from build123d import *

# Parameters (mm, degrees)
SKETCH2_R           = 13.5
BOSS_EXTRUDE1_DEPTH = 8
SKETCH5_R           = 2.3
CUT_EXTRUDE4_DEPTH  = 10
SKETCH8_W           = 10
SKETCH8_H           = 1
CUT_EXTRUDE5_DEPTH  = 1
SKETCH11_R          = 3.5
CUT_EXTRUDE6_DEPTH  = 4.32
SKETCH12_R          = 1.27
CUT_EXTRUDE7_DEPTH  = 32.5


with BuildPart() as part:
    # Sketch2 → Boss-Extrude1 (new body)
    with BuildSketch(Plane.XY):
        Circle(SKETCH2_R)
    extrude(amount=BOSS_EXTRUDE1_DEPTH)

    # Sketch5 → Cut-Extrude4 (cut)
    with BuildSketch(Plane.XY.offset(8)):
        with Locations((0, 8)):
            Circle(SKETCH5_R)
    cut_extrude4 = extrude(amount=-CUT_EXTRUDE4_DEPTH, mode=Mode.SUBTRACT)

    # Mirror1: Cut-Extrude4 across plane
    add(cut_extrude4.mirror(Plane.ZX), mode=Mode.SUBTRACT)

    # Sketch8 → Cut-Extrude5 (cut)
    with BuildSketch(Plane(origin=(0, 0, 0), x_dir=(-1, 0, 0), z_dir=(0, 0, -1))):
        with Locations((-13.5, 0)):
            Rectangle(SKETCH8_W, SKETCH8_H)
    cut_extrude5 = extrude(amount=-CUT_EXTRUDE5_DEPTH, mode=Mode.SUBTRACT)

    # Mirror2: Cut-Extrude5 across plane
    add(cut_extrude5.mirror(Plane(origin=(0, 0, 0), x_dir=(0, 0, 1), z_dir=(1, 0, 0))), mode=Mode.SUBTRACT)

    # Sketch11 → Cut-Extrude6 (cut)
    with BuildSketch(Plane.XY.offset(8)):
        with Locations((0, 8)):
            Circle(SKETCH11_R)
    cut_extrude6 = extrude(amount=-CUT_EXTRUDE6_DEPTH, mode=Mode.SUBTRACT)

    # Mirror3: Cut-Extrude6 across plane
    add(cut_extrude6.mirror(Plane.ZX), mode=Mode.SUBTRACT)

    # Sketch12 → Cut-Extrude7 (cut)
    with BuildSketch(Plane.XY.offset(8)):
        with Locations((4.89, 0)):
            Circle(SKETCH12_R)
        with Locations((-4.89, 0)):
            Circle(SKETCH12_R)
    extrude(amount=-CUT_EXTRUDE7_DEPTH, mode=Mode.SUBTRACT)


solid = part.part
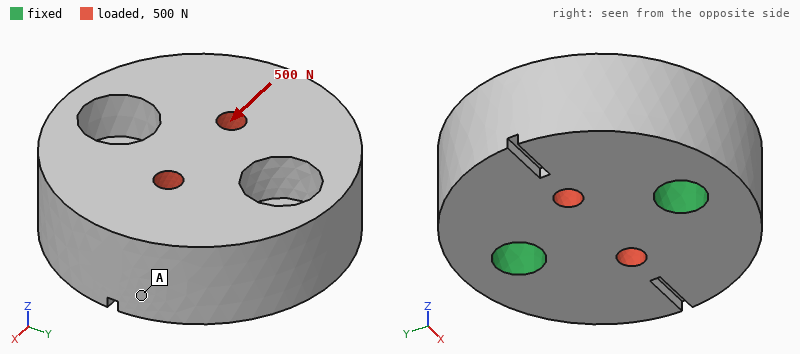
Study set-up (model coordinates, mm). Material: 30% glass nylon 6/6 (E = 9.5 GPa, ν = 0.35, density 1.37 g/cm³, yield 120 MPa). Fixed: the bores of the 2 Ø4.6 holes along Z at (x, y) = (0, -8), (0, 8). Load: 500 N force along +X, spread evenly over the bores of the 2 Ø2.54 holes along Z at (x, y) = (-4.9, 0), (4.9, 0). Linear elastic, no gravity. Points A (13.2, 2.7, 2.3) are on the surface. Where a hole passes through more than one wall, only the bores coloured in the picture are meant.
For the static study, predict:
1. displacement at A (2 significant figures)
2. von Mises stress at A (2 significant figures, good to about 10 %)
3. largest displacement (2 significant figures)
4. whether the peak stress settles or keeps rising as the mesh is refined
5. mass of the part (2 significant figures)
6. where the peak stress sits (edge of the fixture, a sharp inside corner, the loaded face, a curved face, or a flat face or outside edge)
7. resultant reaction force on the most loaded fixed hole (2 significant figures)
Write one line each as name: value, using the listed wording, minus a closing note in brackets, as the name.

displacement at A: 14 µm
von Mises stress at A: 2.3 MPa
largest displacement: 18 µm
whether the peak stress settles or keeps rising as the mesh is refined: keeps rising
mass of the part: 5.5 g
where the peak stress sits: edge of the fixture
resultant reaction force on the most loaded fixed hole: 250 N
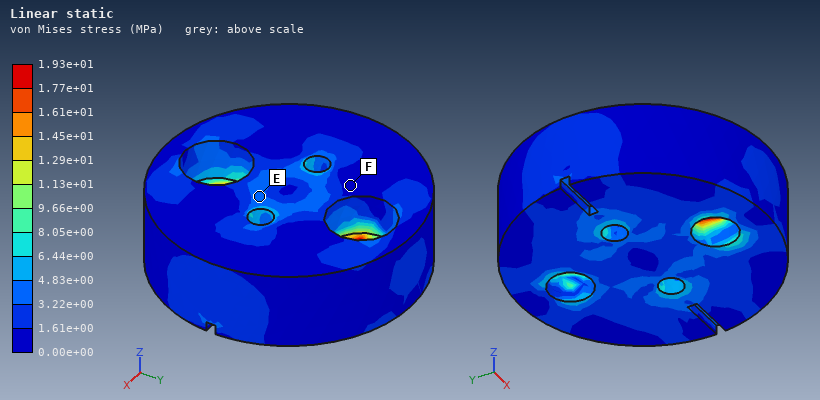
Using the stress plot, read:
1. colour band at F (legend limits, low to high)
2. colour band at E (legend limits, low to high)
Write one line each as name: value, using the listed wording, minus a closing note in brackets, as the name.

colour band at F: 0.00e+00 to 1.61e+00 MPa
colour band at E: 3.22e+00 to 4.83e+00 MPa
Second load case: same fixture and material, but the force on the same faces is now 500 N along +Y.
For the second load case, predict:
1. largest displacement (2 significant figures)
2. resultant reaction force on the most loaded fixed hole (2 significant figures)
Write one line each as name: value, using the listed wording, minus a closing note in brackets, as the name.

largest displacement: 5.0 µm
resultant reaction force on the most loaded fixed hole: 260 N
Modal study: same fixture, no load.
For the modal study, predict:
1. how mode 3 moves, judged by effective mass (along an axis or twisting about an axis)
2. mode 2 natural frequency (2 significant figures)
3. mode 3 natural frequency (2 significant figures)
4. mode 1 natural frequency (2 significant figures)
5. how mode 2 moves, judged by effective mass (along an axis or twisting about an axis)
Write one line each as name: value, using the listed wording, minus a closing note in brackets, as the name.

how mode 3 moves, judged by effective mass: twisting about Z
mode 2 natural frequency: 16 kHz
mode 3 natural frequency: 23 kHz
mode 1 natural frequency: 9300 Hz
how mode 2 moves, judged by effective mass: along Z
